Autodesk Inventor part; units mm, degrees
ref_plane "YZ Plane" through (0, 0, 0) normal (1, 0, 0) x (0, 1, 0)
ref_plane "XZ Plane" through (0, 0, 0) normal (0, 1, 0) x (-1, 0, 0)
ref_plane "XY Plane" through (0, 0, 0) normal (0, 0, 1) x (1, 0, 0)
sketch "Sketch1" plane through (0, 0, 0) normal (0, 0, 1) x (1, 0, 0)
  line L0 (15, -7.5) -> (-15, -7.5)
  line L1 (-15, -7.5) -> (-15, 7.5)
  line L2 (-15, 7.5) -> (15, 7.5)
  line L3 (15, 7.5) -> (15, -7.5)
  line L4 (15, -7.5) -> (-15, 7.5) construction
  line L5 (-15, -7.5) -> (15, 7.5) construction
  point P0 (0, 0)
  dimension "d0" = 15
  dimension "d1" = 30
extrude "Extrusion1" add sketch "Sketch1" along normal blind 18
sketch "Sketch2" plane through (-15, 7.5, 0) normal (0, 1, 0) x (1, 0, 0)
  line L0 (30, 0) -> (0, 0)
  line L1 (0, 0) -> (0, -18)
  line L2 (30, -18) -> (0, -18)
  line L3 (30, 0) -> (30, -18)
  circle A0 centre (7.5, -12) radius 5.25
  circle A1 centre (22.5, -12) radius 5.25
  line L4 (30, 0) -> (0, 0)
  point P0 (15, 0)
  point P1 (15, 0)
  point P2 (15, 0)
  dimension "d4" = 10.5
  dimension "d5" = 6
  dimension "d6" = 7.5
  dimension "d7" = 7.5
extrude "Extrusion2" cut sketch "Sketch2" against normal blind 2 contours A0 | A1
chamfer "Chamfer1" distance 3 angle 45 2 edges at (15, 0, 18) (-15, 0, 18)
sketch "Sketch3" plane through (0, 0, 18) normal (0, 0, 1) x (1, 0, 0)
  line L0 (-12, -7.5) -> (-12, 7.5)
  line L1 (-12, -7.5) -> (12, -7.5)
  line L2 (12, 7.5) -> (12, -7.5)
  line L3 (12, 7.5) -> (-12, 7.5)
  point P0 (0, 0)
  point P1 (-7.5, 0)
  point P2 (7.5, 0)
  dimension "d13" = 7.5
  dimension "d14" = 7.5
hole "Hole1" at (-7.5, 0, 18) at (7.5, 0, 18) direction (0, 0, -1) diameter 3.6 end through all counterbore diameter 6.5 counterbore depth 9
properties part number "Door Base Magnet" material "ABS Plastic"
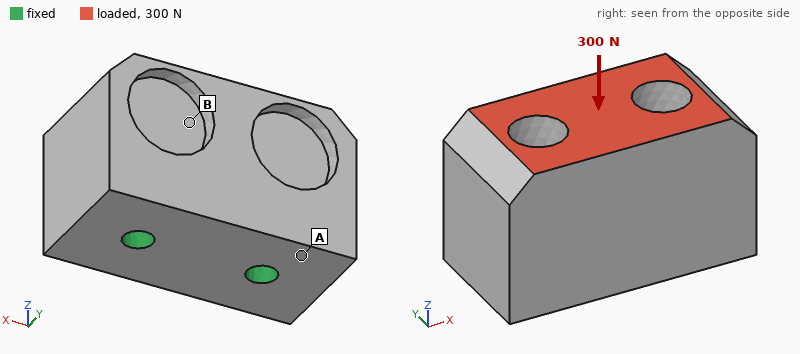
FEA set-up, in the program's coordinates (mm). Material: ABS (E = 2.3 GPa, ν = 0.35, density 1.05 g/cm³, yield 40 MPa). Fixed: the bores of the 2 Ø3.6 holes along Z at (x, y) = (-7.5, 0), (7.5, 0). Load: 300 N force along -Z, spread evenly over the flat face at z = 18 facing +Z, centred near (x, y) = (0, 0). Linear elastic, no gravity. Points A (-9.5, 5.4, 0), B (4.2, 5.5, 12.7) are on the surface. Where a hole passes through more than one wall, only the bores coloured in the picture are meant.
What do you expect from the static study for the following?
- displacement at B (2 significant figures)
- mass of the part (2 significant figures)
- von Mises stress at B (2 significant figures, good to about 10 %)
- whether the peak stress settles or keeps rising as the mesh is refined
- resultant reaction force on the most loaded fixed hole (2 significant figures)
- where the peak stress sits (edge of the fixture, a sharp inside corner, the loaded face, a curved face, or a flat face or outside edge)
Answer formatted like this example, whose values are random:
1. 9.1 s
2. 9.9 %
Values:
1. 7.7 µm
2. 7.2 g
3. 1.7 MPa
4. keeps rising
5. 150 N
6. edge of the fixture
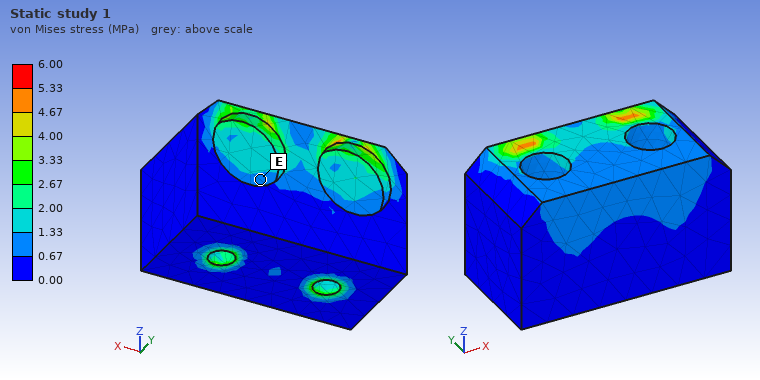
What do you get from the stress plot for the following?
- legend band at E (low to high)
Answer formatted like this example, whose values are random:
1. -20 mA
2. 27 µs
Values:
1. 0.67 to 1.33 MPa
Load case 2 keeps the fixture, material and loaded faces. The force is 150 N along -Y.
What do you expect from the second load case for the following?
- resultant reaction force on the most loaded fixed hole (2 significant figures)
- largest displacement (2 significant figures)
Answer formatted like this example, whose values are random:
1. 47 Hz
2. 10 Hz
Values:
1. 75 N
2. 49 µm
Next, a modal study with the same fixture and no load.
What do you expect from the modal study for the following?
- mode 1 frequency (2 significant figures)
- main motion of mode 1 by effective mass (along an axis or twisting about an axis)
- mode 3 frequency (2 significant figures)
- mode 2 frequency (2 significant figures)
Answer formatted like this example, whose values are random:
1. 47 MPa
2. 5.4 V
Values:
1. 7800 Hz
2. along Y
3. 11 kHz
4. 11 kHz
